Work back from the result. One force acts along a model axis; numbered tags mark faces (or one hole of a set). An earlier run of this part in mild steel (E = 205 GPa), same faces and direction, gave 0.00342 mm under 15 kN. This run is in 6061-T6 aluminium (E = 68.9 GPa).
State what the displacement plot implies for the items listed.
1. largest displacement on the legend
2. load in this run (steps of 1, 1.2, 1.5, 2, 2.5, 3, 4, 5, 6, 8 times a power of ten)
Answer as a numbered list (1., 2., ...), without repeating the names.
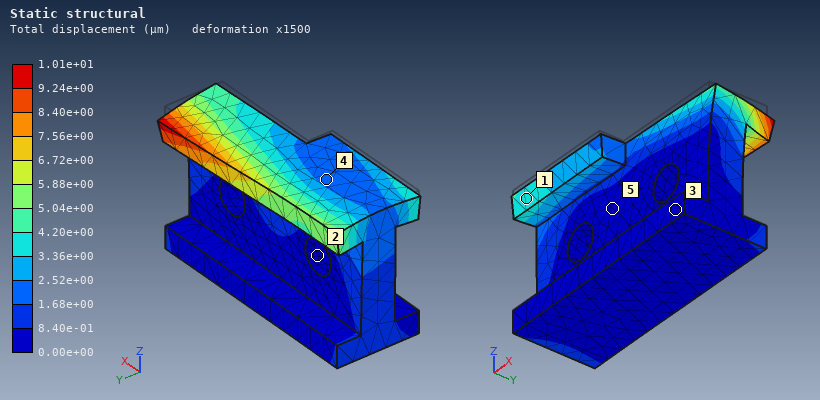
1. 1.01e+01 µm
2. 15 kN
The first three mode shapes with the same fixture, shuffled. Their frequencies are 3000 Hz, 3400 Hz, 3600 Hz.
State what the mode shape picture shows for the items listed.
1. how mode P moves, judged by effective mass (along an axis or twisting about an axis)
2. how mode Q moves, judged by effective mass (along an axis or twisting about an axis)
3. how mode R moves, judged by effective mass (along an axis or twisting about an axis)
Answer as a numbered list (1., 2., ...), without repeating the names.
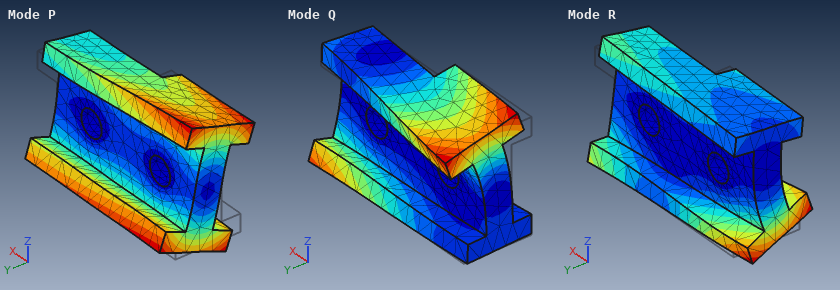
1. twisting about X
2. along Y
3. along Y
